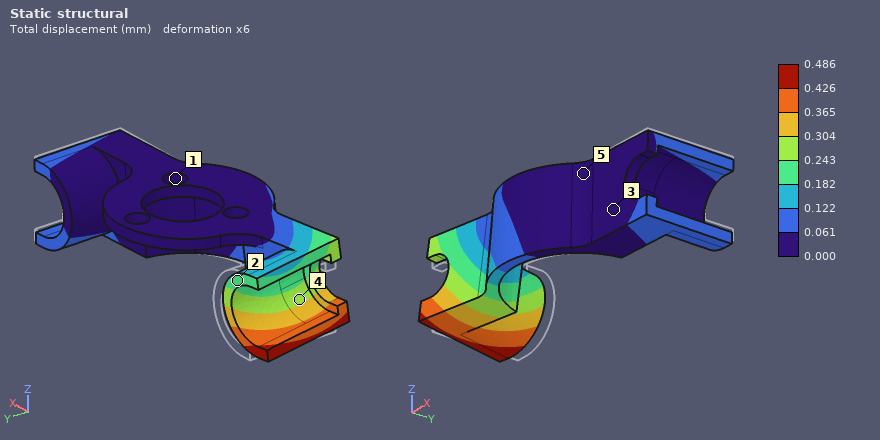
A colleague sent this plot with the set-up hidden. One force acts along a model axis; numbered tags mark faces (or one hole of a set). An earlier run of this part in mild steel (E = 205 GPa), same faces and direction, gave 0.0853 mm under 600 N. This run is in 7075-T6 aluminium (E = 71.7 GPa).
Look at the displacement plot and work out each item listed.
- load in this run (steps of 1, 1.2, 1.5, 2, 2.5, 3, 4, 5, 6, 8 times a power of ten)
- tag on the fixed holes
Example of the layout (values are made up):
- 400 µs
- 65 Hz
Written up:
- 1.2 kN
- 1
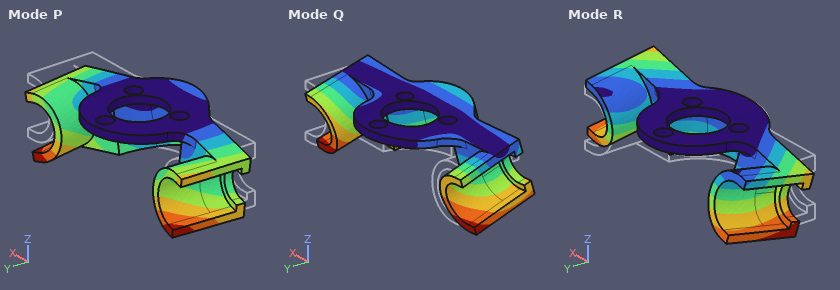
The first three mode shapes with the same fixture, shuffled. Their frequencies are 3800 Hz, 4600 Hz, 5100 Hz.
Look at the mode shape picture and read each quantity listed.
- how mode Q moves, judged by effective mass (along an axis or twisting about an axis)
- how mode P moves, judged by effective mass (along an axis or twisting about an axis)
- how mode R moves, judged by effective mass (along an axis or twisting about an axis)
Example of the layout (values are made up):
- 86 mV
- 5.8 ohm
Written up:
- along Y
- along Z
- along X
